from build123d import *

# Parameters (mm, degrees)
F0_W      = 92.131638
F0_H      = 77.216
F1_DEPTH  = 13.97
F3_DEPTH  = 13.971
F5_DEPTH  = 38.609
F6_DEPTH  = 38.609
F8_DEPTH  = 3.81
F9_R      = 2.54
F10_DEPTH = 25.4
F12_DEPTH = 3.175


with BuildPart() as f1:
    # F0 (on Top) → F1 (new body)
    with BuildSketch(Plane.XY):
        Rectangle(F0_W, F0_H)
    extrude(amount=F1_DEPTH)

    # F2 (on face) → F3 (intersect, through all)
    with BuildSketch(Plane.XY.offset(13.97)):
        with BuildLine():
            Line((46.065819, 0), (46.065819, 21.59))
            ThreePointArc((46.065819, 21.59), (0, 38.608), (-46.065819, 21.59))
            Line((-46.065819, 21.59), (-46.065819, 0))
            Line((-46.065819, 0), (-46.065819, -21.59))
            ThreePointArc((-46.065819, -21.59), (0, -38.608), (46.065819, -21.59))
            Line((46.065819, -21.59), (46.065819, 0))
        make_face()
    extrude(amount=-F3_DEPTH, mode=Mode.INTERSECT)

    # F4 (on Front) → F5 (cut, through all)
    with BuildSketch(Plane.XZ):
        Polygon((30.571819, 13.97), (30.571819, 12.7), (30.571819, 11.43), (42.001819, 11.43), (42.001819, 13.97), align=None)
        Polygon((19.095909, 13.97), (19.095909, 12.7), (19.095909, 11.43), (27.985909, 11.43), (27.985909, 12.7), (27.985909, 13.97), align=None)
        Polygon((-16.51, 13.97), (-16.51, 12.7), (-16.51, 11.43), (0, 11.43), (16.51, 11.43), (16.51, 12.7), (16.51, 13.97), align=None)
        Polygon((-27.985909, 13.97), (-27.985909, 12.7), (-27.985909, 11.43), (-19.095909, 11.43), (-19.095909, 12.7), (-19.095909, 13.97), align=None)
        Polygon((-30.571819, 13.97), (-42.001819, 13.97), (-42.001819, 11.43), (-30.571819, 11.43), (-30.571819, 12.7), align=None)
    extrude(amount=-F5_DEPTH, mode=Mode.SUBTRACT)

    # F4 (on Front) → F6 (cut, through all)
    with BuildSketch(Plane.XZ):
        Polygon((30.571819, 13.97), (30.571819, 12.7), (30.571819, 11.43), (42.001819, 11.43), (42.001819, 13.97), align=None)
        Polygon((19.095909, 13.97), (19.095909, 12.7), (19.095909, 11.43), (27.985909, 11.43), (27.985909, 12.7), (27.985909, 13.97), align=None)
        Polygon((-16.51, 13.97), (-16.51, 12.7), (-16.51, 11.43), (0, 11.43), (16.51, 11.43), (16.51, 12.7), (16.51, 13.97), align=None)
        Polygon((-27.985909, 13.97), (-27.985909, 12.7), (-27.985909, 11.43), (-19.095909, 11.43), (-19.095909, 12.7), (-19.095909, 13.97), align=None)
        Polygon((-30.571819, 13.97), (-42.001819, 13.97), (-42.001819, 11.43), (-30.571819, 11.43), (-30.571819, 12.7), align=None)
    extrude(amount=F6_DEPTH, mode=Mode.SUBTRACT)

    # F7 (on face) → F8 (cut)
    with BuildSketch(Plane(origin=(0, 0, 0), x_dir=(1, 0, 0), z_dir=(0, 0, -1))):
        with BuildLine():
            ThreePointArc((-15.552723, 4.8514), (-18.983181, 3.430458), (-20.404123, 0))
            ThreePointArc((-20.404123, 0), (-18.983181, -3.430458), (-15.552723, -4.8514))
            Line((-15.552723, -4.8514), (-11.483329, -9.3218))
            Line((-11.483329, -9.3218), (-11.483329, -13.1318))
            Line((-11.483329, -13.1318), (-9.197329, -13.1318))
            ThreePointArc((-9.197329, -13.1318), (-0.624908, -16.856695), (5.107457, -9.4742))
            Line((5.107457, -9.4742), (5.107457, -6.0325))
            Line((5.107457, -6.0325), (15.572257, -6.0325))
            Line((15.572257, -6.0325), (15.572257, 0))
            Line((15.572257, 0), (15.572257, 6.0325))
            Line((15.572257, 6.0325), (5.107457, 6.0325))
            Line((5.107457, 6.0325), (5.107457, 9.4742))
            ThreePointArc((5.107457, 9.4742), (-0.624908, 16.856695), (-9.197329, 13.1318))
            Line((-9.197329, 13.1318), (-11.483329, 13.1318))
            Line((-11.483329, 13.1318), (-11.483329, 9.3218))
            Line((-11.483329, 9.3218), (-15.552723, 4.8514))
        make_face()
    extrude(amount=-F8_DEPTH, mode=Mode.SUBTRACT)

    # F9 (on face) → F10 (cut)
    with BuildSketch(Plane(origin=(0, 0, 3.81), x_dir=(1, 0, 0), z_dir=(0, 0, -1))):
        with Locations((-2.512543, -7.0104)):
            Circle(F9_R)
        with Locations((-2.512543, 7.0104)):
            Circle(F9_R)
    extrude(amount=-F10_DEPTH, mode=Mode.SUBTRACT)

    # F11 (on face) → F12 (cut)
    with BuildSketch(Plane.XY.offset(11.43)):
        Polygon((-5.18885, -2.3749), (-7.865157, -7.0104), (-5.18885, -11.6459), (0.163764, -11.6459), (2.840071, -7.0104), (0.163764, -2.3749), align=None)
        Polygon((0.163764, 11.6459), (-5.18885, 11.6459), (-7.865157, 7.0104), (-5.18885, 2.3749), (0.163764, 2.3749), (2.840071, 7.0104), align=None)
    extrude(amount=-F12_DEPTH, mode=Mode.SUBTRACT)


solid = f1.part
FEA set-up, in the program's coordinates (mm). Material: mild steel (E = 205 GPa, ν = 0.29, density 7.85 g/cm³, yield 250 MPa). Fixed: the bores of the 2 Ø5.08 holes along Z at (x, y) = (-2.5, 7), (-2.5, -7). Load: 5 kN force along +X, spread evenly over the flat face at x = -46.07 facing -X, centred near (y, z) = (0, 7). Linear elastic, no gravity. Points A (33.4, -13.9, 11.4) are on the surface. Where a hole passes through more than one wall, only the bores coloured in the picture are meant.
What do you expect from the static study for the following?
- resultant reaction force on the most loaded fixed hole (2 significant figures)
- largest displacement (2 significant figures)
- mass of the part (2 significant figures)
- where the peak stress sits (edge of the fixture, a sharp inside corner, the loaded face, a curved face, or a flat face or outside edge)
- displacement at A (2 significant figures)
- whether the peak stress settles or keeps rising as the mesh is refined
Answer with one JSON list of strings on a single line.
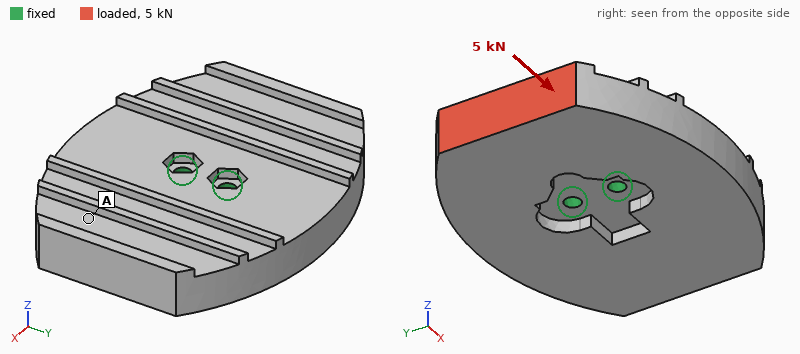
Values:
["2.5 kN", "10.0 µm", "540 g", "edge of the fixture", "4.5 µm", "keeps rising"]
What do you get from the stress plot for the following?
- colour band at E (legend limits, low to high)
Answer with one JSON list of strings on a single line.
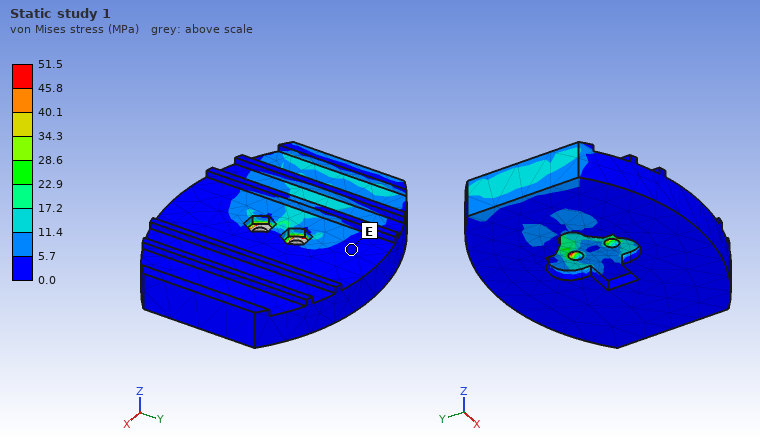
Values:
["0.0 to 5.7 MPa"]
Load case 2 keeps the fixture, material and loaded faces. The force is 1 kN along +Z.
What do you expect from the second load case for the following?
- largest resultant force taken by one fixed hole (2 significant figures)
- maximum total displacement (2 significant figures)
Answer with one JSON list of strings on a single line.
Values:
["500 N", "81 µm"]
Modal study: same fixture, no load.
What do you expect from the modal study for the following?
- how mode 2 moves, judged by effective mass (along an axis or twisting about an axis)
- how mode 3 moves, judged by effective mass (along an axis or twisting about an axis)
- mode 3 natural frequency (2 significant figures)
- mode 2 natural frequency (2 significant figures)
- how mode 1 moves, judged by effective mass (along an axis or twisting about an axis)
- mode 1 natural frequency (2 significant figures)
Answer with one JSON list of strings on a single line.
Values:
["twisting about X", "twisting about Z", "3500 Hz", "3100 Hz", "twisting about Y", "1400 Hz"]
